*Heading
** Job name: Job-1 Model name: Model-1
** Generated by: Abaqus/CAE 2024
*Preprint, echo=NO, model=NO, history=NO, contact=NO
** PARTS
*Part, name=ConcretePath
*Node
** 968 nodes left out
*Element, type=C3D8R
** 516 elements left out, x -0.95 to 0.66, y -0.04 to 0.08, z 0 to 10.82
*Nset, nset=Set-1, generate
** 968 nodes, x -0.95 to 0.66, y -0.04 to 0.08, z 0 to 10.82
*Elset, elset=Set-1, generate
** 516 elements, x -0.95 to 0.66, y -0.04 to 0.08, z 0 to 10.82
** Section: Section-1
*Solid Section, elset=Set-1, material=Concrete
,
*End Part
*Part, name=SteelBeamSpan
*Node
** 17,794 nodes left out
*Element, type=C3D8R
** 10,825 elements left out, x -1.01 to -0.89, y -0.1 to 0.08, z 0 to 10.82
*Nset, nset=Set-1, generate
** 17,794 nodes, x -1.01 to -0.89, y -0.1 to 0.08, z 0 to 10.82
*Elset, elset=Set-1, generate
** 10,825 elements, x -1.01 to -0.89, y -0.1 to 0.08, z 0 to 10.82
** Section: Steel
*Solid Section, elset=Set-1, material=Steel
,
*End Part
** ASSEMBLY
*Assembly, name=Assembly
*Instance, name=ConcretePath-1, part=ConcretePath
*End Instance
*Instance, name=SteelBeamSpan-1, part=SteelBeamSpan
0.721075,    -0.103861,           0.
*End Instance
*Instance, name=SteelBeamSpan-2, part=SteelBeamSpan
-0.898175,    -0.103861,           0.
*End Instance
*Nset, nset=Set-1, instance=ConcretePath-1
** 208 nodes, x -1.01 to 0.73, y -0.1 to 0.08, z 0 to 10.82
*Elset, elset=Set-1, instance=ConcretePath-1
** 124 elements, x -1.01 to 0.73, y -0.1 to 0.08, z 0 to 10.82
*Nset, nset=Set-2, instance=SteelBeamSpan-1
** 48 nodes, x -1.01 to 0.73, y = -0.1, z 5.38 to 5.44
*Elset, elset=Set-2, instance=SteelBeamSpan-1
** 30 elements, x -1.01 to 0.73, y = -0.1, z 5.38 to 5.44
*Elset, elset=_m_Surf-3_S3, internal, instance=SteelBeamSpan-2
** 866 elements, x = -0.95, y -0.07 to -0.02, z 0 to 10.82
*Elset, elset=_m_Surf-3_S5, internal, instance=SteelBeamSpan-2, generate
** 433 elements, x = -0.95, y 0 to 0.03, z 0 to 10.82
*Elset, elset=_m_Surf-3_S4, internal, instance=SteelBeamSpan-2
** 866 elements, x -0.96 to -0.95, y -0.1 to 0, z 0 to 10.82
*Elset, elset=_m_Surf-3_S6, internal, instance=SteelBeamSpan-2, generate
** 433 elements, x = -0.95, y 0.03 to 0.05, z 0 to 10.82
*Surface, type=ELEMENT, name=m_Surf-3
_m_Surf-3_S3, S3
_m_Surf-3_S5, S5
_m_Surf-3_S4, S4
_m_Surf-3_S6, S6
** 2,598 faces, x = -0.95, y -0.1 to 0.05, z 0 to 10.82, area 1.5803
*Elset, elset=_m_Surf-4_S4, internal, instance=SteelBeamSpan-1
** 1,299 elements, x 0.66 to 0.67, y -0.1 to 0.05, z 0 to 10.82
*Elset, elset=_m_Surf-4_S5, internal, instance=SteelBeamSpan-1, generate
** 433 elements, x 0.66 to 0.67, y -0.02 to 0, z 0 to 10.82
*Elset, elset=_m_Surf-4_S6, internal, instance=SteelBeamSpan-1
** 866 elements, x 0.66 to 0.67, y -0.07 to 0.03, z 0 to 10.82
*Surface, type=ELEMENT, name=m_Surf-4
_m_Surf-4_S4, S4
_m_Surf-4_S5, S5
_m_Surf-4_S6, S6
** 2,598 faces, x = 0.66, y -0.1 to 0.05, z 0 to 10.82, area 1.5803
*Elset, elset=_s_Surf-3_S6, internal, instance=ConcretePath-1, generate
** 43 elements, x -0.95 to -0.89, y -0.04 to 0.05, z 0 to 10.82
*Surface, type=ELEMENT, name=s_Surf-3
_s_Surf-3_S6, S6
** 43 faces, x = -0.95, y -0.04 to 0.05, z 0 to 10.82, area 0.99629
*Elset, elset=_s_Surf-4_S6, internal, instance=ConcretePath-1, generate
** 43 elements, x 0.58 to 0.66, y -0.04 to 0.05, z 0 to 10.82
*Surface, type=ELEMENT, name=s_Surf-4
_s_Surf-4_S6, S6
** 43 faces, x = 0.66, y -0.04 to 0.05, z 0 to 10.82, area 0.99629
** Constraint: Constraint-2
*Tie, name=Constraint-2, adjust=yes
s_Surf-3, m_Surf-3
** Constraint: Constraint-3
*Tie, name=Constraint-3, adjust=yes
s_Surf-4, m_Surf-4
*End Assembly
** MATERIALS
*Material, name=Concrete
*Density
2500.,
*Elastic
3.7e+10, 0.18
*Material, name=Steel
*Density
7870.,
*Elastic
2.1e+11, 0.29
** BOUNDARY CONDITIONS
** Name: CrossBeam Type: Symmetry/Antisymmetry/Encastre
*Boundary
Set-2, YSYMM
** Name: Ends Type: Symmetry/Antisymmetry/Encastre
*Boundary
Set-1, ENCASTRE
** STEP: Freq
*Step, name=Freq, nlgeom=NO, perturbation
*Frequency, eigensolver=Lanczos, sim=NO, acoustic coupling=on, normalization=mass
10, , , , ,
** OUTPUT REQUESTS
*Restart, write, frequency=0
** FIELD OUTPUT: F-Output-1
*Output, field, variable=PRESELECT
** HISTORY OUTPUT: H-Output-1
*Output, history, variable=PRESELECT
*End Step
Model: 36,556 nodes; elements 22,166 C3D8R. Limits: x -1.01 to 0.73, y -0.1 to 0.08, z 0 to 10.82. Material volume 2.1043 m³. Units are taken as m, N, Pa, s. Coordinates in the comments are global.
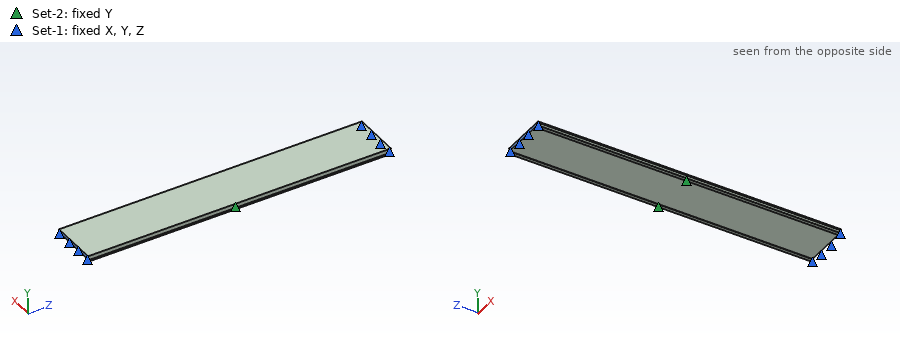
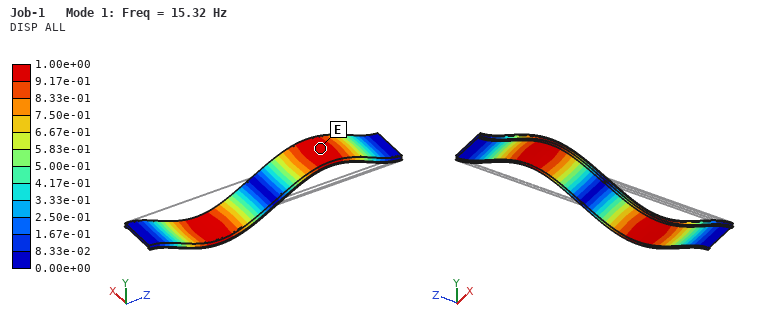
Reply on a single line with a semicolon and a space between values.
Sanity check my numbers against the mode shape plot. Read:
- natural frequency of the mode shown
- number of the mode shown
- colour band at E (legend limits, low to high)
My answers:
15.32 Hz; 1; 9.17e-01 to 1.00e+00
